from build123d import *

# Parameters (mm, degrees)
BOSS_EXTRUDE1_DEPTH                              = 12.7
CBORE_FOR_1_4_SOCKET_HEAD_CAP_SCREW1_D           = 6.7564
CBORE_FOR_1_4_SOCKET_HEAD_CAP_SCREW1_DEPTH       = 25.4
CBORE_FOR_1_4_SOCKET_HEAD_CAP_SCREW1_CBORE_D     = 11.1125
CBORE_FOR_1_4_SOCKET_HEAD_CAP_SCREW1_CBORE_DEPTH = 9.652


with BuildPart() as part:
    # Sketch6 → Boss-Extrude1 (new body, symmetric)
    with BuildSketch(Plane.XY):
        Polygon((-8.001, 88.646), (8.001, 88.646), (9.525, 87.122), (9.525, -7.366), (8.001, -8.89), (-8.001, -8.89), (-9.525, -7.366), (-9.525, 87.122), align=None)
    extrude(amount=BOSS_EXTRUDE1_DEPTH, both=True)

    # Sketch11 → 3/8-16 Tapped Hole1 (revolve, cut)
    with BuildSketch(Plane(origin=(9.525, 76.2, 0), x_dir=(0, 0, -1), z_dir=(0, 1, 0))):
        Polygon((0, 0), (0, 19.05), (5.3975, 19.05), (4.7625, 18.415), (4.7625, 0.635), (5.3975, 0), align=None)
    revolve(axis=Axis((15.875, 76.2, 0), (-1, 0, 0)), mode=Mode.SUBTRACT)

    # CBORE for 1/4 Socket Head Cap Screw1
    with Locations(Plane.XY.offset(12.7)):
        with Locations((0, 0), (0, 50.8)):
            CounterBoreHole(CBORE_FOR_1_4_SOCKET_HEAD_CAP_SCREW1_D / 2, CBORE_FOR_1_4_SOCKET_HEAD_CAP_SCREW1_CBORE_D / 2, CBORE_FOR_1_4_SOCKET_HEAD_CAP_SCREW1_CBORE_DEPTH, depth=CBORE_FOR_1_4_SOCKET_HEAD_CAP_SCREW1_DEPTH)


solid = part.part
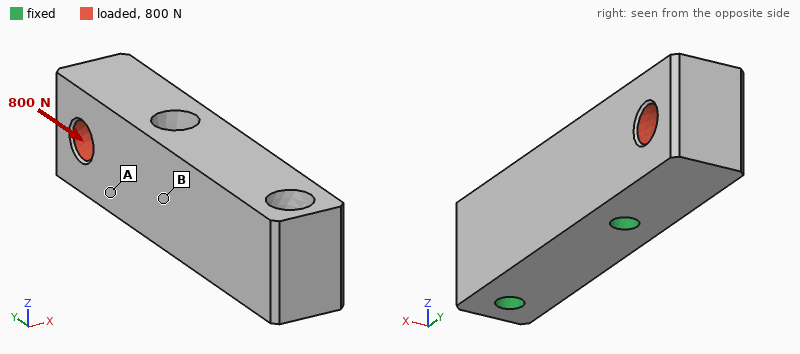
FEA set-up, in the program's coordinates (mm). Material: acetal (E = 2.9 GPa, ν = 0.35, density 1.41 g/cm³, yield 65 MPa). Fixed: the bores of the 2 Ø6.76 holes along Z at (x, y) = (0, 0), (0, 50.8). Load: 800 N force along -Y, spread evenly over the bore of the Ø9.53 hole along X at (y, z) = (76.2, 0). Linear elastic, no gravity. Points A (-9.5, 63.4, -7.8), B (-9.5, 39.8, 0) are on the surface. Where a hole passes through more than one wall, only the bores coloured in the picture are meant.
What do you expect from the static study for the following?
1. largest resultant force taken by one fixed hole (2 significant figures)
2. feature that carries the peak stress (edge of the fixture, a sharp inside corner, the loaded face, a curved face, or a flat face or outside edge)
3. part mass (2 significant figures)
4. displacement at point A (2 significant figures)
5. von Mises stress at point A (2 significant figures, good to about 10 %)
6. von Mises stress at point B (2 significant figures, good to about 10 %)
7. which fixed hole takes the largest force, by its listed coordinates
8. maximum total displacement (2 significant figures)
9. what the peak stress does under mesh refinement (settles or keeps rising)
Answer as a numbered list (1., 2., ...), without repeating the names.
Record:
1. 710 N
2. edge of the fixture
3. 60 g
4. 9.1 µm
5. 1.5 MPa
6. 0.52 MPa
7. (0, 50.8)
8. 39 µm
9. keeps rising
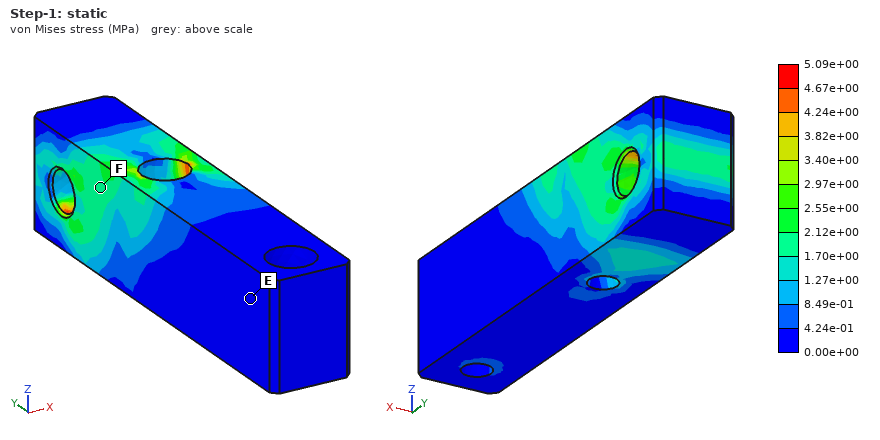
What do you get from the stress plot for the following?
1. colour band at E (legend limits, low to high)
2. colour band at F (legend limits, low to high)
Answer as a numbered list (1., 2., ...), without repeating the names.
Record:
1. 0.00e+00 to 4.24e-01 MPa
2. 1.70e+00 to 2.12e+00 MPa
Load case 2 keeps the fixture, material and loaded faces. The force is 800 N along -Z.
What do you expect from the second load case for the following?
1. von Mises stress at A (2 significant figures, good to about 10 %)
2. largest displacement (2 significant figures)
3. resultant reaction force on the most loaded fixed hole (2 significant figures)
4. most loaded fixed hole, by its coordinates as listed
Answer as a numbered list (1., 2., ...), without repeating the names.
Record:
1. 4.2 MPa
2. 0.28 mm
3. 970 N
4. (0, 50.8)
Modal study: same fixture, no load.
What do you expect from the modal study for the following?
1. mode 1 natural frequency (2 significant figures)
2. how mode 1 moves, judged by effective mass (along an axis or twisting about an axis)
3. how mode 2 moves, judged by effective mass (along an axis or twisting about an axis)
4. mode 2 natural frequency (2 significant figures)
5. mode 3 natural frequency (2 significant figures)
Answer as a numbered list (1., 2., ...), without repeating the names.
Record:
1. 2100 Hz
2. along X
3. along Z
4. 2500 Hz
5. 4200 Hz
